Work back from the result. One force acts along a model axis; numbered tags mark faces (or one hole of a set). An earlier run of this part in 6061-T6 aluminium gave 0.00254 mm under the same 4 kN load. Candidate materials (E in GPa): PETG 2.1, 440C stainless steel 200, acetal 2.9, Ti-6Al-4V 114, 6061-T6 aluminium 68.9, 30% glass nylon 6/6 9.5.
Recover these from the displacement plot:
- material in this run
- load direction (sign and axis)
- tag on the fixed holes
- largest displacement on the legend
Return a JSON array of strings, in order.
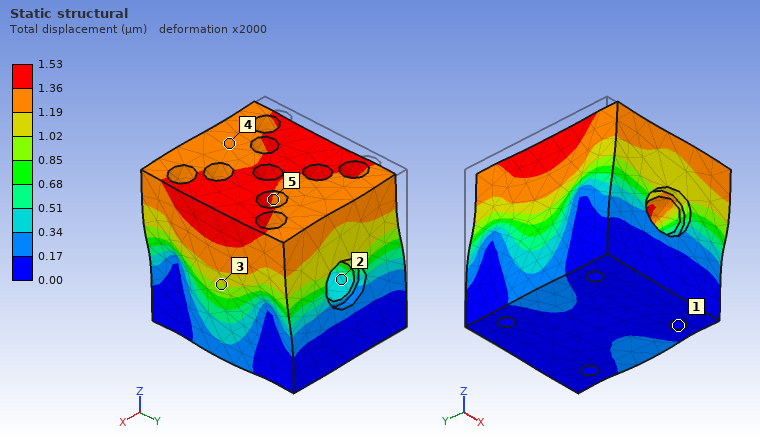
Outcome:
["Ti-6Al-4V", "+X", "1", "1.53 µm"]
